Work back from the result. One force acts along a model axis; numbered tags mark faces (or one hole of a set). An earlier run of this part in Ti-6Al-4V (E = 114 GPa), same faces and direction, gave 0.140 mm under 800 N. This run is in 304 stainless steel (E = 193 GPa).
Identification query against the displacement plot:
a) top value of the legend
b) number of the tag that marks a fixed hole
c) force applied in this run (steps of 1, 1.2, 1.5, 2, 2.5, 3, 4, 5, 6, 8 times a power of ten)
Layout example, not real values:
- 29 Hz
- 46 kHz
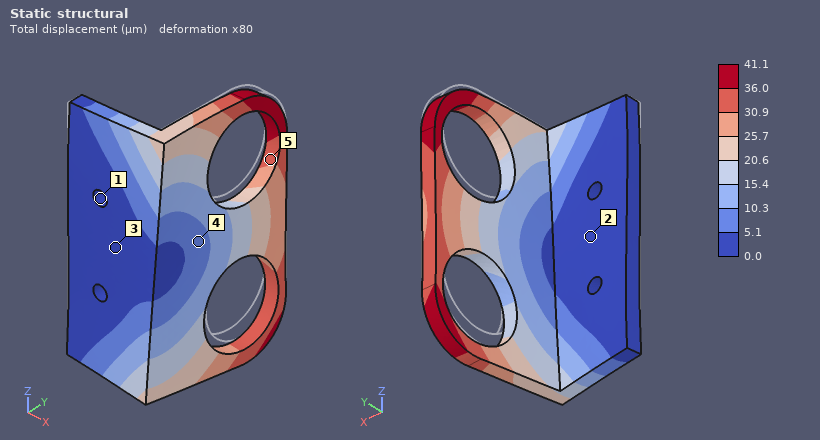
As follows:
- 41.1 µm
- 1
- 400 N
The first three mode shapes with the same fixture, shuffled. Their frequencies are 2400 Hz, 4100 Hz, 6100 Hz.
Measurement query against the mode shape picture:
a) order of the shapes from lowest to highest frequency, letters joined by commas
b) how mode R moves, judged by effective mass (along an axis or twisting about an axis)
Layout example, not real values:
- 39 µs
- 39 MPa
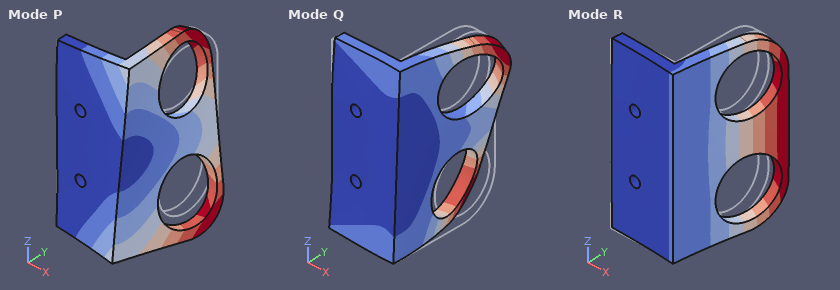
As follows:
- R, P, Q
- along X
